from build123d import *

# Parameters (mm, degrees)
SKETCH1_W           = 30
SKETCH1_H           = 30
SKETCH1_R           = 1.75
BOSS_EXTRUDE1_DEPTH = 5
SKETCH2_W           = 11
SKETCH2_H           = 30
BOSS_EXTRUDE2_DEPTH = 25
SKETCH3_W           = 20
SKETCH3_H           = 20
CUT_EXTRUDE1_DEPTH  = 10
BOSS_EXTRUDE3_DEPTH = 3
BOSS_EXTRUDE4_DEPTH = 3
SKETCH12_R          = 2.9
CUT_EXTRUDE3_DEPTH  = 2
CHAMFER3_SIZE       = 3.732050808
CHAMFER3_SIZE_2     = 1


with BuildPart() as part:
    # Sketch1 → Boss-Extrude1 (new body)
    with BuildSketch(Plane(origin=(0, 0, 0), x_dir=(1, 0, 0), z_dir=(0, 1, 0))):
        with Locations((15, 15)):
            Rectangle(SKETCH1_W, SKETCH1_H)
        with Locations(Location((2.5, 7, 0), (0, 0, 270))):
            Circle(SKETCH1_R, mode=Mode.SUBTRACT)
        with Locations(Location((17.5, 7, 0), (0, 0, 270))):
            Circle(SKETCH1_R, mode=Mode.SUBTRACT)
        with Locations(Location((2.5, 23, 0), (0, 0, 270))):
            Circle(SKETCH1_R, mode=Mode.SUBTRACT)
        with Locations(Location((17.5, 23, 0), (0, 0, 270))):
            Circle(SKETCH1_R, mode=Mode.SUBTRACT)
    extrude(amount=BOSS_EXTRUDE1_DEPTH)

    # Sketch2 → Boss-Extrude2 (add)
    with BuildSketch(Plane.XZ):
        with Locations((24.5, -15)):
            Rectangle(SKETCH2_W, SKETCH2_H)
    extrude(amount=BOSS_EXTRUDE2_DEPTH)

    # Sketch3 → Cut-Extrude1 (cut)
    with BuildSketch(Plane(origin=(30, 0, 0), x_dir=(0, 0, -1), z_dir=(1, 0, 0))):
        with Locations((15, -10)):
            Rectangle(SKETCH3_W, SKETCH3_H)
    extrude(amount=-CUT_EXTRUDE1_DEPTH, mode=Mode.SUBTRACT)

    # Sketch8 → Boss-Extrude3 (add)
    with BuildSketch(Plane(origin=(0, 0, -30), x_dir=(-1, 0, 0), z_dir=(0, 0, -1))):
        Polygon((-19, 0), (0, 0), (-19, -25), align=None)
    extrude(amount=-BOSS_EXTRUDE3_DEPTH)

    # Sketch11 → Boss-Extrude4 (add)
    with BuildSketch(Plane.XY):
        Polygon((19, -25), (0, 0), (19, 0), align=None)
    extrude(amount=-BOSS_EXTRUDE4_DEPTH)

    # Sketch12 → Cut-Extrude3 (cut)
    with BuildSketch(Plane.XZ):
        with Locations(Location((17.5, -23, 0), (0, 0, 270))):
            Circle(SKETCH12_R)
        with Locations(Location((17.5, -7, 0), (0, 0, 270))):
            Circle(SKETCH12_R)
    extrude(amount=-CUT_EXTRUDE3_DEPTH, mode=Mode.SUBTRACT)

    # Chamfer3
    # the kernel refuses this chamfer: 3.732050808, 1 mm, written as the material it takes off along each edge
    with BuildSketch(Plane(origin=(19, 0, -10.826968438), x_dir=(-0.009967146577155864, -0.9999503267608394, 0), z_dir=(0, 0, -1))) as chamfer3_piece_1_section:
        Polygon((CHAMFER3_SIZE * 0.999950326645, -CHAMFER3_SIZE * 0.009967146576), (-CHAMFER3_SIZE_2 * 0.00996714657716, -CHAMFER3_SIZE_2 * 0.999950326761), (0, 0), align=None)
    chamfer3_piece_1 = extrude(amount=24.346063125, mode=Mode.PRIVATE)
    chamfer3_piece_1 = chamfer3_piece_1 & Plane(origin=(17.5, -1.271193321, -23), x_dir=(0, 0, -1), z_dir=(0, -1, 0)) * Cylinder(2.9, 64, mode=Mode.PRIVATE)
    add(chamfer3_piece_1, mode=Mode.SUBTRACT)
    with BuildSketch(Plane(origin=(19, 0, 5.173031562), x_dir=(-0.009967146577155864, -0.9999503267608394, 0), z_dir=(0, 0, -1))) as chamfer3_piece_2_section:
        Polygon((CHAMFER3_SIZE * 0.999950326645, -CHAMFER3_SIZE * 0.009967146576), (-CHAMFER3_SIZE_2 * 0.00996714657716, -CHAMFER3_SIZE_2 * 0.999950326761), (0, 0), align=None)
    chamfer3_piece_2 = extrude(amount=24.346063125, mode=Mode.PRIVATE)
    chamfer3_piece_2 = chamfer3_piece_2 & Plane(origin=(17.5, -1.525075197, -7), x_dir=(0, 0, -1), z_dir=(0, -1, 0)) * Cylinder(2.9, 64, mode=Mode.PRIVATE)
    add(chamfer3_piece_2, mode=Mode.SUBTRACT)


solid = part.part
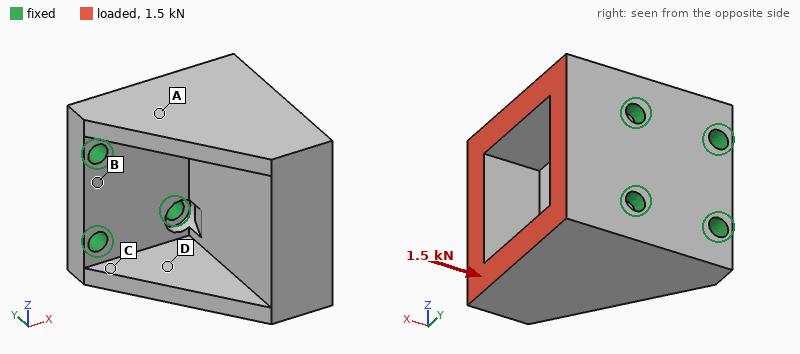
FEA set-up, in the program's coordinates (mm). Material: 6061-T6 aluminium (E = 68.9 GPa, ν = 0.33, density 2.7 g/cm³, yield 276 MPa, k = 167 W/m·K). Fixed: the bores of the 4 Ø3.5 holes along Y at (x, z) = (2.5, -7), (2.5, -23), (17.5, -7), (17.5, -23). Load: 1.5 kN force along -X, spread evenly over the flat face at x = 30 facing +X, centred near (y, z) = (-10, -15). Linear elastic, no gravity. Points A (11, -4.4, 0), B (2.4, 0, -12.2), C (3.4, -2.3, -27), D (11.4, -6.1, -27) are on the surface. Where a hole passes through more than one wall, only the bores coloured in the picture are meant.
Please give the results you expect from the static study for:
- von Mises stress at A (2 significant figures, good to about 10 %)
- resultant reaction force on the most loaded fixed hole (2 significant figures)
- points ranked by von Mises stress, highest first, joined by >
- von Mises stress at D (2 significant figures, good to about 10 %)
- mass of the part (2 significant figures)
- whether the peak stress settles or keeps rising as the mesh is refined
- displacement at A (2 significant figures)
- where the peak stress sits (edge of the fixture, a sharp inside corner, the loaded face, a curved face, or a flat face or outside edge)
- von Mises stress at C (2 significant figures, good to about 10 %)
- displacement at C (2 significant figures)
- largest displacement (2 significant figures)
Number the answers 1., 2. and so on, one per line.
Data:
1. 16 MPa
2. 760 N
3. C > D > A > B
4. 23 MPa
5. 27 g
6. keeps rising
7. 7.5 µm
8. edge of the fixture
9. 45 MPa
10. 7.3 µm
11. 41 µm
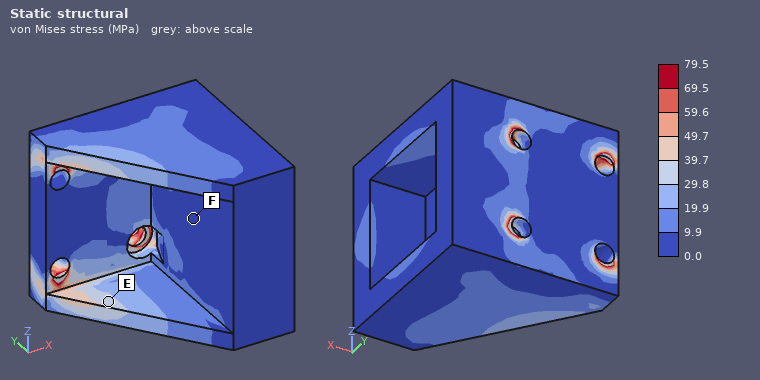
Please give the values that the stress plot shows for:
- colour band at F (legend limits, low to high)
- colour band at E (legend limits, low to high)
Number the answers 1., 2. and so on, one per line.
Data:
1. 0.0 to 9.9 MPa
2. 29.8 to 39.7 MPa
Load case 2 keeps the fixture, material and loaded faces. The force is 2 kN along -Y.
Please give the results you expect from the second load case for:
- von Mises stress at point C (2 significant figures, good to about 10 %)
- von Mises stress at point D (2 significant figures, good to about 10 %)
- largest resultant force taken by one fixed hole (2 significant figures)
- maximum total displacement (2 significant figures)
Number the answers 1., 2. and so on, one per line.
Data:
1. 52 MPa
2. 21 MPa
3. 1.7 kN
4. 67 µm
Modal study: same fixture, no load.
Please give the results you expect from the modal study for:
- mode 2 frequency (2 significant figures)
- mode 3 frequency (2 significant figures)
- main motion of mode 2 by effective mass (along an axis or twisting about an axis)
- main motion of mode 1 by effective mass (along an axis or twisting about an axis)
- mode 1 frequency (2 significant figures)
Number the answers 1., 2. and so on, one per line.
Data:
1. 8100 Hz
2. 13 kHz
3. along X
4. along Z
5. 7700 Hz
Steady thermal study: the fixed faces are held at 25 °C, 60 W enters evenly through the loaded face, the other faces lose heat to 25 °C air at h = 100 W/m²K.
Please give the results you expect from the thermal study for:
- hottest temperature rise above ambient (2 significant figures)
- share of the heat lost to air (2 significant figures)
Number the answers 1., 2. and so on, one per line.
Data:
1. 35 K
2. 14 %
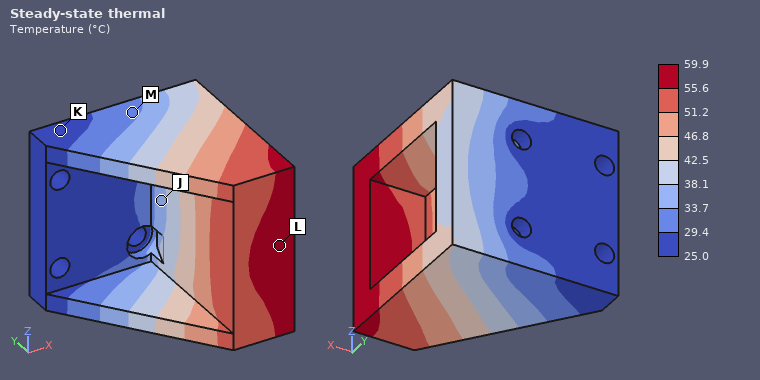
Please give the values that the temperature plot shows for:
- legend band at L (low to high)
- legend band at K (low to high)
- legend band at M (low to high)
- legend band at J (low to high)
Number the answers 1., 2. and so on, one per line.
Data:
1. 55.6 to 59.9 °C
2. 25.0 to 29.4 °C
3. 29.4 to 33.7 °C
4. 33.7 to 38.1 °C
